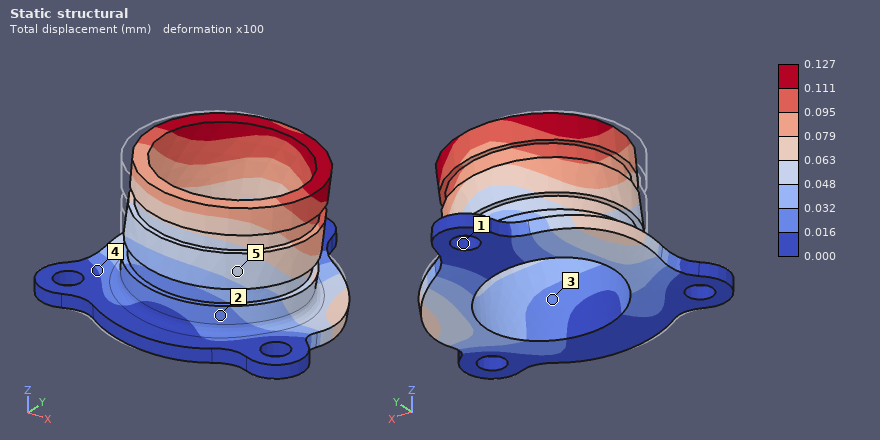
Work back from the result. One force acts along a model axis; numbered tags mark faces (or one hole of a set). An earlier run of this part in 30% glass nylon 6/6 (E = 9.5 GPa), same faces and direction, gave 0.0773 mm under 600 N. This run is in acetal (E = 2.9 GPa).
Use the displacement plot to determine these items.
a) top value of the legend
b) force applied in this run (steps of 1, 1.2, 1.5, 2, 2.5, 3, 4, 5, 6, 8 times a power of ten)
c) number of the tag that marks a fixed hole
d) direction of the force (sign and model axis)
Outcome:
0.127 mm
300 N
1
+X
